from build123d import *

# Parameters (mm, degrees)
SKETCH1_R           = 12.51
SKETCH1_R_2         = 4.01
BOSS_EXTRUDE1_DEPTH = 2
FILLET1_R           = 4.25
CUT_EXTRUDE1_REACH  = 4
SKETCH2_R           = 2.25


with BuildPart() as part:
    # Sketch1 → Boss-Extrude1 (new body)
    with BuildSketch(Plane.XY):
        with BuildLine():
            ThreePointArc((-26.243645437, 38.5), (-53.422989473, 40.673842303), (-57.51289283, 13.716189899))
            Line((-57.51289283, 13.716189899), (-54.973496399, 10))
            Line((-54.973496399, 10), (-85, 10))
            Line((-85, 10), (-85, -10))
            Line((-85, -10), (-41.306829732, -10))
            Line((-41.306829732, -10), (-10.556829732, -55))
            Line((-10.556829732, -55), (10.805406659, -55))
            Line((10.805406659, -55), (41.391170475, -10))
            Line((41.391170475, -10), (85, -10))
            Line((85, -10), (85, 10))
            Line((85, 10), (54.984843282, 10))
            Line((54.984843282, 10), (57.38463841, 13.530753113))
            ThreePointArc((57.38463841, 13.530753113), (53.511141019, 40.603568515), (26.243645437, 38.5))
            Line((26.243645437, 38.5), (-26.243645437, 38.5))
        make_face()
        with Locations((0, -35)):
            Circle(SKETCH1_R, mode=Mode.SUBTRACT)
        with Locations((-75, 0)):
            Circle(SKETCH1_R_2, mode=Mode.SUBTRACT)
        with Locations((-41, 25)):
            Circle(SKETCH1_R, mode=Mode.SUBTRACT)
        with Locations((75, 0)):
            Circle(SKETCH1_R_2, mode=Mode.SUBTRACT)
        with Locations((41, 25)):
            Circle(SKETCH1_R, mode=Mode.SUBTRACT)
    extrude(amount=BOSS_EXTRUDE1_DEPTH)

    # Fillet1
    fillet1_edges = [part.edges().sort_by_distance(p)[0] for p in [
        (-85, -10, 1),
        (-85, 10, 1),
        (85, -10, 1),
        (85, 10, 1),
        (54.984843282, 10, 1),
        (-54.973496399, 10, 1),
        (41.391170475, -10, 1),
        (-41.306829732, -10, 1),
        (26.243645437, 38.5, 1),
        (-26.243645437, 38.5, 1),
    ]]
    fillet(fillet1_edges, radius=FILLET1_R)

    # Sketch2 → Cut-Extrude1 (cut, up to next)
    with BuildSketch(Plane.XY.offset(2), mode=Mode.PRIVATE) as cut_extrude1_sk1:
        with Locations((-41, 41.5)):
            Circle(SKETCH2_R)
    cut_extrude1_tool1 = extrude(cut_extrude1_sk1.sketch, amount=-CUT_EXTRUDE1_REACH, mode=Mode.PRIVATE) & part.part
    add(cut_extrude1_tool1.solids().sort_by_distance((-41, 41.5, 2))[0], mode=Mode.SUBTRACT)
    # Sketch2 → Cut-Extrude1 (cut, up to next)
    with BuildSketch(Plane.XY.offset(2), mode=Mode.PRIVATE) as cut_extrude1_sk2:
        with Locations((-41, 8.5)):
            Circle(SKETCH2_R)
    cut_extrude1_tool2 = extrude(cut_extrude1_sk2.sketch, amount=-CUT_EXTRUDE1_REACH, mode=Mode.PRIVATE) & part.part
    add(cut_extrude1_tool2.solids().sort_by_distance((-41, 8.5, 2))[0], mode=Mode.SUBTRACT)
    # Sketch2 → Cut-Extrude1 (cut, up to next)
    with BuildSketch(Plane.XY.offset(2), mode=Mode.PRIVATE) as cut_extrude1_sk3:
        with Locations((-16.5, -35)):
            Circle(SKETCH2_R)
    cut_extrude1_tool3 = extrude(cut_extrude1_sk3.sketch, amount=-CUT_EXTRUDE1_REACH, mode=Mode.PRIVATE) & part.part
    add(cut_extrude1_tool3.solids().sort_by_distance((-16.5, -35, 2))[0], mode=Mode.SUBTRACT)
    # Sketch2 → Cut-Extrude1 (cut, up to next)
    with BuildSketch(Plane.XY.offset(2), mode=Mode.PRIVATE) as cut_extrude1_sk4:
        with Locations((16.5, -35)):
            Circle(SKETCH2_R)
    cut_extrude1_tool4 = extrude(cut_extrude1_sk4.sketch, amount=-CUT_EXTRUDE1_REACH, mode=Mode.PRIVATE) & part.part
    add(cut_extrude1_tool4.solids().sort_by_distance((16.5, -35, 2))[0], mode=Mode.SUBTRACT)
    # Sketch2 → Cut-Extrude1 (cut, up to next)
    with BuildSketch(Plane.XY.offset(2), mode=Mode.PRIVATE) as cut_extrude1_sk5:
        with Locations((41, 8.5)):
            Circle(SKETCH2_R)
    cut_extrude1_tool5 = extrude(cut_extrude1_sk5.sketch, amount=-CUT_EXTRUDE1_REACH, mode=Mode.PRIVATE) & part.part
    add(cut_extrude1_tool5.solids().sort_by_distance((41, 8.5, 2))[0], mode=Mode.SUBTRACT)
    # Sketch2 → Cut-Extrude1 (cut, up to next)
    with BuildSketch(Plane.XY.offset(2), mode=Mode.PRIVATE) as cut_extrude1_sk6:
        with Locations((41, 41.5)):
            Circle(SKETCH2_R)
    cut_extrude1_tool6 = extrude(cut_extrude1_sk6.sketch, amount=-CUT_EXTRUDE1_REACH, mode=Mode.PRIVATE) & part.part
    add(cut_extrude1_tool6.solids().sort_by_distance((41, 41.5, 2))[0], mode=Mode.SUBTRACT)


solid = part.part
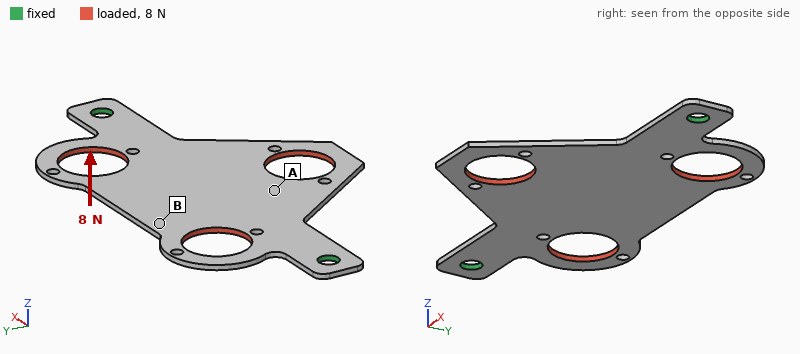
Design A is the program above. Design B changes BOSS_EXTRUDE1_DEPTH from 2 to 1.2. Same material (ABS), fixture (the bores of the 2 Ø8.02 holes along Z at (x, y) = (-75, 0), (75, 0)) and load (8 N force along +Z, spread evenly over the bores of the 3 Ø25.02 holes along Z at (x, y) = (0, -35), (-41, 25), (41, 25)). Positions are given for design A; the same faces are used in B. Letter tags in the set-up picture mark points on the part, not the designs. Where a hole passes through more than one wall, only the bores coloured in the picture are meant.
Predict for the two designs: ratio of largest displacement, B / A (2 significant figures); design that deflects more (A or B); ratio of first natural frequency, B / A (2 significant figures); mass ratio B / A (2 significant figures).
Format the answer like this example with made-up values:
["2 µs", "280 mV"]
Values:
["4.6", "B", "0.61", "0.60"]
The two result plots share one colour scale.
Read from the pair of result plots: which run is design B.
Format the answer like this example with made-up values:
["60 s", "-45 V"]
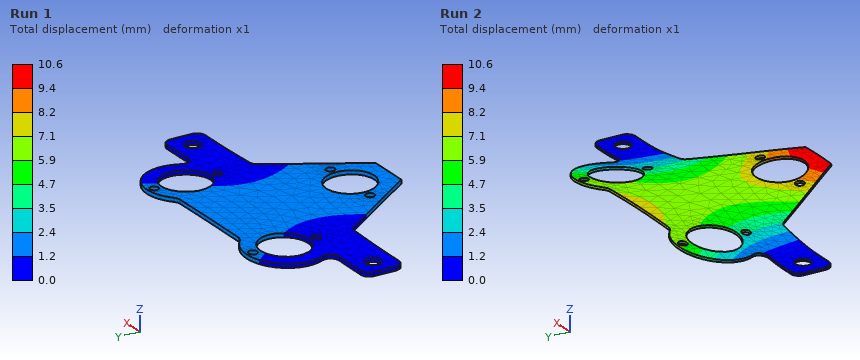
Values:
["Run 2"]
